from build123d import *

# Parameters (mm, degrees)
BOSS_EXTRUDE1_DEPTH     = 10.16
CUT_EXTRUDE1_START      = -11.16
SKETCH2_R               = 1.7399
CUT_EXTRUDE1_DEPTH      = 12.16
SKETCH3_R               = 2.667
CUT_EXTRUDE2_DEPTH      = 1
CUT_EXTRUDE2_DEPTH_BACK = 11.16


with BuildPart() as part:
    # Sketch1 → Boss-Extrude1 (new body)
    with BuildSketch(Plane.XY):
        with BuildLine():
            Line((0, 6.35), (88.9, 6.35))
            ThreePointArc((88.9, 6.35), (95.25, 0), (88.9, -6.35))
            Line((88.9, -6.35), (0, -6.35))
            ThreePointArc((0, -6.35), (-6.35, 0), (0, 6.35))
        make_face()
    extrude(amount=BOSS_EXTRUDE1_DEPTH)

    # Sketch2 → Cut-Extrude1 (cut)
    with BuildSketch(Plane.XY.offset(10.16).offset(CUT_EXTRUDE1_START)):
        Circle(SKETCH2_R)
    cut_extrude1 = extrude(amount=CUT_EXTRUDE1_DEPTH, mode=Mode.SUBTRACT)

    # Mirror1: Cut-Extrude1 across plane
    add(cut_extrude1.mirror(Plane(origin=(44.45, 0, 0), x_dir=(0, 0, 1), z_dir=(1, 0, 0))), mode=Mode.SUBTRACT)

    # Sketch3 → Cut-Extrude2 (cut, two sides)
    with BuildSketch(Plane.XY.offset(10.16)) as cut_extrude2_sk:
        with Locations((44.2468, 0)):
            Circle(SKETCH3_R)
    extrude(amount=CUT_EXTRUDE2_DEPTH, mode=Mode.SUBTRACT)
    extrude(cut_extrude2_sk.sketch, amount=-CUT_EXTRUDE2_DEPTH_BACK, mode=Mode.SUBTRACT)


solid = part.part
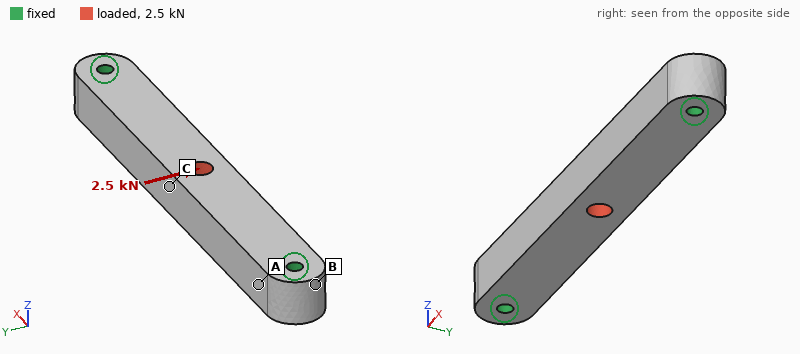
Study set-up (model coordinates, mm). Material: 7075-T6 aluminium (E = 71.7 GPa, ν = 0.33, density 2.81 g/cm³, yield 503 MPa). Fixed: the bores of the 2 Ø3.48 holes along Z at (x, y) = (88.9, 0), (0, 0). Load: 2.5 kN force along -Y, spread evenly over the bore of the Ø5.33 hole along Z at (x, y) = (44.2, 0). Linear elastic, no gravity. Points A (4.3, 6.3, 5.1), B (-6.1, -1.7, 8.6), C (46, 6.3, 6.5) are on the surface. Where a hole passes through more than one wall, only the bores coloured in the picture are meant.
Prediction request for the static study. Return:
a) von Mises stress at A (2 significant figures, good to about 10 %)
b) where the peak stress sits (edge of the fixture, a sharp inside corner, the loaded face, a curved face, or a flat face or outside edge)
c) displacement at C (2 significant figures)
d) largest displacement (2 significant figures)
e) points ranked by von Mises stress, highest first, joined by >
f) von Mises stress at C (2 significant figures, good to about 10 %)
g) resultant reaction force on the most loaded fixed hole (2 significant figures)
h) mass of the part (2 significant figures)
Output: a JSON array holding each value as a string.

["63 MPa", "edge of the fixture", "0.13 mm", "0.13 mm", "C > A > B", "120 MPa", "1.3 kN", "35 g"]
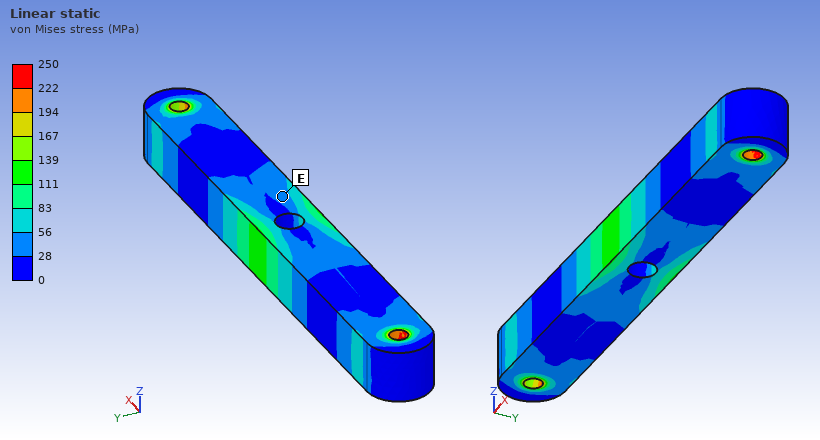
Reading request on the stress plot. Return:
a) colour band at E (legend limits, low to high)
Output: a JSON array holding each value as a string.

["28 to 56 MPa"]
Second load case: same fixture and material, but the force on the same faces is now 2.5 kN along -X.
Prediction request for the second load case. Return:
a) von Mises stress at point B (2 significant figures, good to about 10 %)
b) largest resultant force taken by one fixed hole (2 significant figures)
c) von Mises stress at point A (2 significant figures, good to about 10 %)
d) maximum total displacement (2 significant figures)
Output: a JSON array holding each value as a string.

["3.4 MPa", "1.3 kN", "5.8 MPa", "6.4 µm"]
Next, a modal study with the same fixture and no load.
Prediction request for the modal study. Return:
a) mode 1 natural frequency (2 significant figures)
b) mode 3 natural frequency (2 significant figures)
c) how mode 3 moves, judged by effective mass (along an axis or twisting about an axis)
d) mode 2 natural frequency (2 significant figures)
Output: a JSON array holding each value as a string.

["6000 Hz", "15 kHz", "twisting about Y", "6000 Hz"]
